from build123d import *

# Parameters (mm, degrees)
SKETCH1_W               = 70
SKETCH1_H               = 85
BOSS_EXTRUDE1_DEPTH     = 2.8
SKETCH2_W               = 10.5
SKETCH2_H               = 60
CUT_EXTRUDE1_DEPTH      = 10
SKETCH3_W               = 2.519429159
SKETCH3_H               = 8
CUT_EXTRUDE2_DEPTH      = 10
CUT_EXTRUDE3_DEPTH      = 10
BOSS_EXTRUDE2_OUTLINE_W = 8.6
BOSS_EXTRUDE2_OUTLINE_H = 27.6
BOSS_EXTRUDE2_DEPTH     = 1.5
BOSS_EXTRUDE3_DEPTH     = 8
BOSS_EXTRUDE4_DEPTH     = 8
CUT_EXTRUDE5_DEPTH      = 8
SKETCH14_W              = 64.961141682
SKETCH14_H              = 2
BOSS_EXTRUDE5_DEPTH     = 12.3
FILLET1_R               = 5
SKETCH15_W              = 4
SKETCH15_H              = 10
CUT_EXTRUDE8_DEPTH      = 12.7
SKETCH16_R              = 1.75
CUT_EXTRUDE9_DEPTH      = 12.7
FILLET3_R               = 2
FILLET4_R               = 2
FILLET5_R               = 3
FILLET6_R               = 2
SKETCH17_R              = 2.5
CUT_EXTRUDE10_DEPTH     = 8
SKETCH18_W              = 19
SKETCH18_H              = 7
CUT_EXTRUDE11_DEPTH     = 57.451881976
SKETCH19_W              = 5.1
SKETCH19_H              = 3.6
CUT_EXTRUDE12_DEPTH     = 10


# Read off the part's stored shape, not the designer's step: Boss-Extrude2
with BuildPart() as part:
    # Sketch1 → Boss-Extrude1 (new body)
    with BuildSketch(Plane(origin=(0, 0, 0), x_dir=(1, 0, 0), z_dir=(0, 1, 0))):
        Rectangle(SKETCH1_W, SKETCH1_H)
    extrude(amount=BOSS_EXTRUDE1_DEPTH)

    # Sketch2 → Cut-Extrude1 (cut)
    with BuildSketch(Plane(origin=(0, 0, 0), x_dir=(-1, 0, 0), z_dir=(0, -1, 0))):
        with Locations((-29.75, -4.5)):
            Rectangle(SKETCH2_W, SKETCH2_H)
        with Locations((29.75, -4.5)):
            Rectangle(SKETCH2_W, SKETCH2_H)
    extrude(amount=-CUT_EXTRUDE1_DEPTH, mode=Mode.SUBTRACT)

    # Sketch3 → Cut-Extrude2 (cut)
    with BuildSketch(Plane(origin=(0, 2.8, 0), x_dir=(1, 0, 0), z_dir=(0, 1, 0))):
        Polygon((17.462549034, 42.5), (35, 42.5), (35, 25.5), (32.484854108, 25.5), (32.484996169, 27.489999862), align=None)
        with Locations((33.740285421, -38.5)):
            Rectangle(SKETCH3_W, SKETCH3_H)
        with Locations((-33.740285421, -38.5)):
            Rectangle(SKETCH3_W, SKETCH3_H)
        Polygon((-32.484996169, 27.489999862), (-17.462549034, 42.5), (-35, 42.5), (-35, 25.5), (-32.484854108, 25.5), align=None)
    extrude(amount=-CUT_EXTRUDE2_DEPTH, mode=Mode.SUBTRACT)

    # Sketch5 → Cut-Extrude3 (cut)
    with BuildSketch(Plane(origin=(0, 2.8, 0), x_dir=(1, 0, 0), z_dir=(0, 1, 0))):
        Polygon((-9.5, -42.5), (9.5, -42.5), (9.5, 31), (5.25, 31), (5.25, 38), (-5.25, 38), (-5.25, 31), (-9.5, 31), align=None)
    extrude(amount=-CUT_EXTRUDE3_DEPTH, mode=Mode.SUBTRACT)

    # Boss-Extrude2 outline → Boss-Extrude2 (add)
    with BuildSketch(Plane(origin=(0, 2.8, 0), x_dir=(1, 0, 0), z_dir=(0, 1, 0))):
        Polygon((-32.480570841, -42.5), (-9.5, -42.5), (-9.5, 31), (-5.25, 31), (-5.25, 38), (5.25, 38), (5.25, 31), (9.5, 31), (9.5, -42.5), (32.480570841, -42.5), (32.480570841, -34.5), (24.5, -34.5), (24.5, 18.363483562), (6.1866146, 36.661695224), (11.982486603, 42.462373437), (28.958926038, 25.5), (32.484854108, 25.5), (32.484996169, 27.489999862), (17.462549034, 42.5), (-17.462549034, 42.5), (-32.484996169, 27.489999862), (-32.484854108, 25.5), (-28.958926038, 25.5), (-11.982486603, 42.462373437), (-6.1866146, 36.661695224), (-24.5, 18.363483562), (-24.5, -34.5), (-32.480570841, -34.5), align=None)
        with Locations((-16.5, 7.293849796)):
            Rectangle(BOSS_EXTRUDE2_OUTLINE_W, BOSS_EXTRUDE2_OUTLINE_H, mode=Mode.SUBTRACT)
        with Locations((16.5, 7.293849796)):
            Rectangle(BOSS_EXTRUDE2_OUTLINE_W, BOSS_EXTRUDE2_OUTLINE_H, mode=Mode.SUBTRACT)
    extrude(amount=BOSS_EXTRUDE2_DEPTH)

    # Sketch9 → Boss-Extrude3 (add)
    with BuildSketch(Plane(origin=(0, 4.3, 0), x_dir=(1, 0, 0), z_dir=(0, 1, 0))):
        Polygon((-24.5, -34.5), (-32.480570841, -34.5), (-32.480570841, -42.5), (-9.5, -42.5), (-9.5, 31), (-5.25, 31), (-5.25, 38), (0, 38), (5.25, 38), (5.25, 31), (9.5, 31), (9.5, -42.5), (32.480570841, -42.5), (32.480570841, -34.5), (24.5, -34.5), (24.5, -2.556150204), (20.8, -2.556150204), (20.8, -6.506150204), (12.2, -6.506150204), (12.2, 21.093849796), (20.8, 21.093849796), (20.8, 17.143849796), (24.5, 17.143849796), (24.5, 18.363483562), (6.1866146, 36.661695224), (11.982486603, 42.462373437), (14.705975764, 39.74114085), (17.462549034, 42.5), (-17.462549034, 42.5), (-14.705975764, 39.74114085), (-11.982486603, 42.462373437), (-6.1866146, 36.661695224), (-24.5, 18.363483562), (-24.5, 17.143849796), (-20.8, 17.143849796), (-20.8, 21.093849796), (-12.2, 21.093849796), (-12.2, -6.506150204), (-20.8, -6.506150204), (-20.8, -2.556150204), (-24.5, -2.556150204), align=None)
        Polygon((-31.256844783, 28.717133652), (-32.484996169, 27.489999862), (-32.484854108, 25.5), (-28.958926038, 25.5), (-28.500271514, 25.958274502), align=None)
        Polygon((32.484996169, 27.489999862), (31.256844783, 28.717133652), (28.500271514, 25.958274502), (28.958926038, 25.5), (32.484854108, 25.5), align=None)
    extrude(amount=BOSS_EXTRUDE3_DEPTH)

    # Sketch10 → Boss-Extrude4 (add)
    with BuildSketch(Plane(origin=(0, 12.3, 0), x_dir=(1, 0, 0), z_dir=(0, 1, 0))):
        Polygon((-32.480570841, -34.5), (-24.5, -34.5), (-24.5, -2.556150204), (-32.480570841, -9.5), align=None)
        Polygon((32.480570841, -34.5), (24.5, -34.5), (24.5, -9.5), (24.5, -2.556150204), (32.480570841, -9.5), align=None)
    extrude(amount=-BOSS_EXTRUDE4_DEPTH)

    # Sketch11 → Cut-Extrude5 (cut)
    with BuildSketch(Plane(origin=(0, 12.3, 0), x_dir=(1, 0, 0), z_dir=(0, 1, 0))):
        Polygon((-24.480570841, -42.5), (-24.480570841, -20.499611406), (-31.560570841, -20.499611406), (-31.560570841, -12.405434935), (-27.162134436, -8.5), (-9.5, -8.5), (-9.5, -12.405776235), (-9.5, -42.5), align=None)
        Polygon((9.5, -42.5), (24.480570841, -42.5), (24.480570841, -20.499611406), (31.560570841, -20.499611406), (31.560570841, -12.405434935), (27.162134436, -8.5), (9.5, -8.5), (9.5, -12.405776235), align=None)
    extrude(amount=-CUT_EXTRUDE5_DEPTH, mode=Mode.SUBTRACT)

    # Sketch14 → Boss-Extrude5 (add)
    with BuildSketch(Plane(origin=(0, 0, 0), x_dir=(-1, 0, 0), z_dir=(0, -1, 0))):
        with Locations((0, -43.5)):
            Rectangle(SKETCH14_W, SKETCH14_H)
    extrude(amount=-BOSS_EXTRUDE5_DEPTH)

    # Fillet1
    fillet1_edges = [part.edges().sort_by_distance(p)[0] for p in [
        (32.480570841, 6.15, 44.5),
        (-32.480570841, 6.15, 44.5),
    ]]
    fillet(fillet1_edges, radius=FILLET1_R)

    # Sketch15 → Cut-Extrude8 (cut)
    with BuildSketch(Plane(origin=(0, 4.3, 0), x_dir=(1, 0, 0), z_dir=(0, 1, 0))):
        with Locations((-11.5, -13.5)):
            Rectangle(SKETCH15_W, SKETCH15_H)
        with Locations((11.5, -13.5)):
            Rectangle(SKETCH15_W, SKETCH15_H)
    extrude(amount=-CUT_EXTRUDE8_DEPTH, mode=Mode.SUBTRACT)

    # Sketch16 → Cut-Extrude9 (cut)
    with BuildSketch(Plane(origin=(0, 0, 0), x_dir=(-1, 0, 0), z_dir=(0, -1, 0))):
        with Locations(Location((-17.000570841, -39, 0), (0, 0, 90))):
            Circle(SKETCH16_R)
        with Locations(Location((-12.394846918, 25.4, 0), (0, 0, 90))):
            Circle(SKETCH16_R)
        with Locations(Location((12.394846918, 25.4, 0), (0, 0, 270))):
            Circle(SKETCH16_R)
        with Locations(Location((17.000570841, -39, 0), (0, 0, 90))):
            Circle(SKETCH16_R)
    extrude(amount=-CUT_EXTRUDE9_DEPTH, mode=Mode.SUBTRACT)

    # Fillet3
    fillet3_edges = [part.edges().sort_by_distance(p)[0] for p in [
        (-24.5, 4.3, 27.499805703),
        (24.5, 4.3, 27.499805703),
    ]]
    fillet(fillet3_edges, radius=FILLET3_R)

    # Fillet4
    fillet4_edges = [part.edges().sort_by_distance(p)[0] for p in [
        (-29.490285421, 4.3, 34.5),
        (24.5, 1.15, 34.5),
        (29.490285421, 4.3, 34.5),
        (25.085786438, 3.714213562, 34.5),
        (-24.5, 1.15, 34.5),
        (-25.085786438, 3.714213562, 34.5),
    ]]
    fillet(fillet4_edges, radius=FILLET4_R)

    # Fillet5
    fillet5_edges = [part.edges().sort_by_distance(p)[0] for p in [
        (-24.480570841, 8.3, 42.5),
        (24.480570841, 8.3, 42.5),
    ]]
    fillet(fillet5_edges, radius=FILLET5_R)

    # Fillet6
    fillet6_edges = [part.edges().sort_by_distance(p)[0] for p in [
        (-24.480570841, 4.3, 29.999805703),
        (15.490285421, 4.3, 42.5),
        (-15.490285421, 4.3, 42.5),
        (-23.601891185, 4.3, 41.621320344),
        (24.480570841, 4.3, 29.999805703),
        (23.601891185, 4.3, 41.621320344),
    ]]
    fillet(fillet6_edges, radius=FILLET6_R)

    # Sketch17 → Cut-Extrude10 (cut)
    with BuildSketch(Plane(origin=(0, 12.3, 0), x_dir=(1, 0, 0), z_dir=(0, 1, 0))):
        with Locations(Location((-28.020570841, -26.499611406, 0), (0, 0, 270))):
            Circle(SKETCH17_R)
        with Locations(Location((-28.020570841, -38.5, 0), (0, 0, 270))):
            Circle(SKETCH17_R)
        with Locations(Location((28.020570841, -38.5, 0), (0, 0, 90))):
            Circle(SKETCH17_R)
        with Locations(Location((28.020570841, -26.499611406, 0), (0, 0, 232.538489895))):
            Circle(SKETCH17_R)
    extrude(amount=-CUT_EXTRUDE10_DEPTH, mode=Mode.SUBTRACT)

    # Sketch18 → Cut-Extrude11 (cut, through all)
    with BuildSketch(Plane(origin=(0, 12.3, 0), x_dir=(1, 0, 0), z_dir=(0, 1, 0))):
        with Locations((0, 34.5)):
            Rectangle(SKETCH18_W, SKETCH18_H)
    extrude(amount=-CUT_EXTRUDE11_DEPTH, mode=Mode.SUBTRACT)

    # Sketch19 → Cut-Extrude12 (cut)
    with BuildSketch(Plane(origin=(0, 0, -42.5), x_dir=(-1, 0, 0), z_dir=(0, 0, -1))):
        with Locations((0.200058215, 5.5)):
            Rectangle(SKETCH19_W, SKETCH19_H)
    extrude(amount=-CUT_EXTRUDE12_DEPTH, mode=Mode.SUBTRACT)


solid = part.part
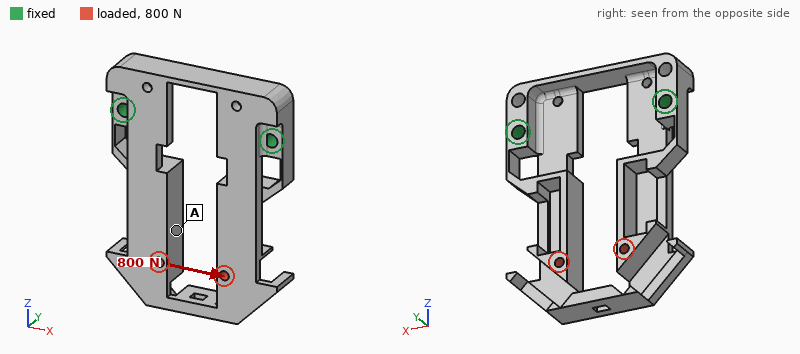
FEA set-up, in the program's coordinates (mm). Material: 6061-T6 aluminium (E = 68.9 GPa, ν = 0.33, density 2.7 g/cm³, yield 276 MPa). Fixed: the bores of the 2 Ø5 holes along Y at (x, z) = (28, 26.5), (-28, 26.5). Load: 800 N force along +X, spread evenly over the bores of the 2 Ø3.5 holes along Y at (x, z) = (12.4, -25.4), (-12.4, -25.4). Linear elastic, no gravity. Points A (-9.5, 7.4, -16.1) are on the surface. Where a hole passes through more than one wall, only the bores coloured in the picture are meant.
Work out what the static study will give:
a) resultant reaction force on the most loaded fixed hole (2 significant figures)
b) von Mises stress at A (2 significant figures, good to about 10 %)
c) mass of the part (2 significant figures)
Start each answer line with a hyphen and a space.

- 560 N
- 36 MPa
- 51 g
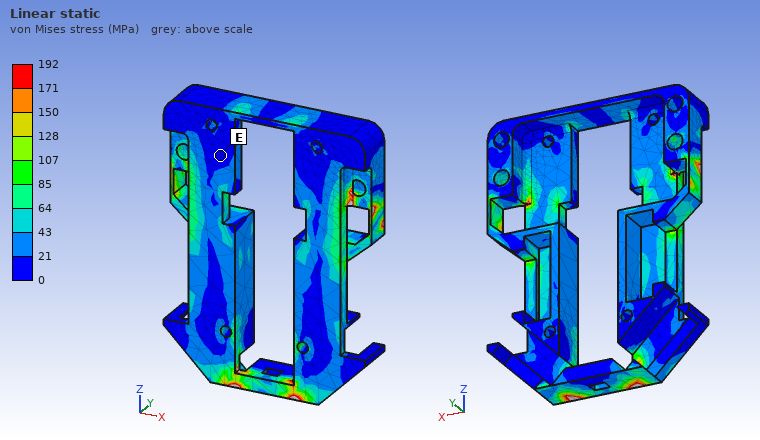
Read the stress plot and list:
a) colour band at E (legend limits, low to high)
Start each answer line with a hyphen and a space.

- 0 to 21 MPa
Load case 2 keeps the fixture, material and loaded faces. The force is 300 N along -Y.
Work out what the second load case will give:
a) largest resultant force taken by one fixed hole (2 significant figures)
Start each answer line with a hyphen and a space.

- 210 N
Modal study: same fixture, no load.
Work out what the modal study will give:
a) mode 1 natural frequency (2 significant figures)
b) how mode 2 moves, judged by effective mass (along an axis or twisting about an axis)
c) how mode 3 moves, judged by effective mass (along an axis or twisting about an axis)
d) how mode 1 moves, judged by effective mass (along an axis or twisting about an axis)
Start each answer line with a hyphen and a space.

- 730 Hz
- along X
- along X
- along Y
